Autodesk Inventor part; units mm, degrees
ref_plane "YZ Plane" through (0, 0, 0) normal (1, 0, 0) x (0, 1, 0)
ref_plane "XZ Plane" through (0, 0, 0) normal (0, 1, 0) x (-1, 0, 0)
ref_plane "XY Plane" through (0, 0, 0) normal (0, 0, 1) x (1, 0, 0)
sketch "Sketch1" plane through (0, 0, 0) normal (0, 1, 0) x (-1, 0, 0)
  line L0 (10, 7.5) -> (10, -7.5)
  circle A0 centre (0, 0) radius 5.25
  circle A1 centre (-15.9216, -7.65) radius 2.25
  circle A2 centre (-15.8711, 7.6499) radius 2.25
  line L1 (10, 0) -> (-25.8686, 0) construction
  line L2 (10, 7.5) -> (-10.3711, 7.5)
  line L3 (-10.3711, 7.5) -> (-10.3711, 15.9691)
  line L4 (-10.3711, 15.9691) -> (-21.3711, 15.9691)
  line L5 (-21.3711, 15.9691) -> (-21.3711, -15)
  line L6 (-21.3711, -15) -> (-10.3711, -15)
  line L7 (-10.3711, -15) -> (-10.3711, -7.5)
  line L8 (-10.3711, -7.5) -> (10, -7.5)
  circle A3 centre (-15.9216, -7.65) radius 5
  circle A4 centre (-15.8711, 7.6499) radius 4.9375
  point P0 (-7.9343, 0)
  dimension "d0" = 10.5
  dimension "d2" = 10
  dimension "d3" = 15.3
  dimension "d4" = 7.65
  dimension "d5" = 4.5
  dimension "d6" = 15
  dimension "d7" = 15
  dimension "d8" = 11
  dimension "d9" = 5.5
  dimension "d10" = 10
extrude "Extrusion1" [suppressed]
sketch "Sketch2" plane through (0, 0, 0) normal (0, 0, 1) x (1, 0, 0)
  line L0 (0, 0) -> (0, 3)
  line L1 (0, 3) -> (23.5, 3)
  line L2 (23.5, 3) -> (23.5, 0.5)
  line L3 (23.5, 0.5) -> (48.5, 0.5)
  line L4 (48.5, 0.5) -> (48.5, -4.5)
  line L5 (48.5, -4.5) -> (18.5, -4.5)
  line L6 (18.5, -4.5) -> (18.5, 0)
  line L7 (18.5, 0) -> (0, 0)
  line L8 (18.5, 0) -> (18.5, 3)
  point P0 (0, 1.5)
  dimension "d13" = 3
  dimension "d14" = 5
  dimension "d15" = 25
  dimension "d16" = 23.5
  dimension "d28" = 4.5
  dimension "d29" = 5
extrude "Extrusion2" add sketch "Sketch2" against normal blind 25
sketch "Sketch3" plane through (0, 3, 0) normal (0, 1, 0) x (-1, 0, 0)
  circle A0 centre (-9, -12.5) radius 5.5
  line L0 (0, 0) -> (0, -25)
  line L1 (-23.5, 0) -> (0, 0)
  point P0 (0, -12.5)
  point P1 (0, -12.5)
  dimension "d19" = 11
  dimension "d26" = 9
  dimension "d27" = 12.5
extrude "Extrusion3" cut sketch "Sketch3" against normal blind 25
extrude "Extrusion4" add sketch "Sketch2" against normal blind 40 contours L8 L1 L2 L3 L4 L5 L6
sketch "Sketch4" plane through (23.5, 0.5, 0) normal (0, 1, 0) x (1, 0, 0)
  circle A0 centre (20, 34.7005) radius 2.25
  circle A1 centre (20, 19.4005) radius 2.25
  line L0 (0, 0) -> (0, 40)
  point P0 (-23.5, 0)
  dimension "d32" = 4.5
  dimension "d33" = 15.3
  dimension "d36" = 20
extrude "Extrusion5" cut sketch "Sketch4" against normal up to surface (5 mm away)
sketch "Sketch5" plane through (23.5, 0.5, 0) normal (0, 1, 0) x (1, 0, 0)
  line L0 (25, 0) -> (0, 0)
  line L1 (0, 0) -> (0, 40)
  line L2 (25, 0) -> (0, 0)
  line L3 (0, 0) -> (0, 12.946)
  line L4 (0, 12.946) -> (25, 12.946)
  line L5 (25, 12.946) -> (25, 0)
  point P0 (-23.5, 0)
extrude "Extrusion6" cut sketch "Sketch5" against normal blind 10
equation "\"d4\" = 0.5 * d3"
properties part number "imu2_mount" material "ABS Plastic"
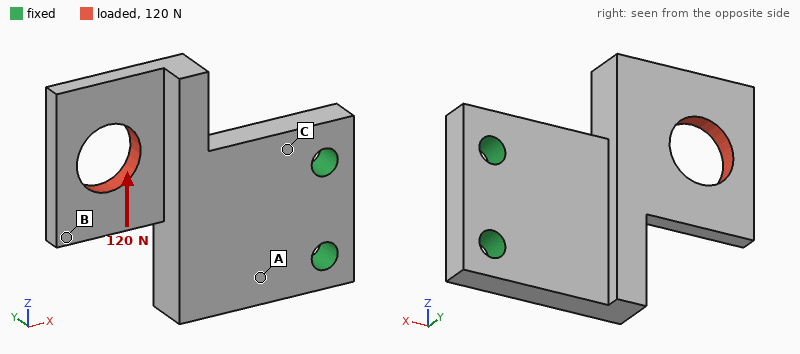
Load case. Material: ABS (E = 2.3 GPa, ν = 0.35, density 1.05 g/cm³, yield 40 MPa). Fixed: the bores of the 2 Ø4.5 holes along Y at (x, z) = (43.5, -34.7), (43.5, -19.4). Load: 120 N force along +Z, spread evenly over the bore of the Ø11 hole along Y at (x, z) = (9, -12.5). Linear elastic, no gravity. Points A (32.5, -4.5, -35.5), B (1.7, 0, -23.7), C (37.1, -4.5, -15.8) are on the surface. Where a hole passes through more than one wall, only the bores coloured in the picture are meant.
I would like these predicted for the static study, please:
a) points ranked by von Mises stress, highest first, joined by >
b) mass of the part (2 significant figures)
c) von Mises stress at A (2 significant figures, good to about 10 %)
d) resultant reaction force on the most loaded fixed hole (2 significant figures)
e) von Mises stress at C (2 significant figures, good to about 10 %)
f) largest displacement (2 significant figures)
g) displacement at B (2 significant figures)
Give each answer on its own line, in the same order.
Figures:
C > A > B
6.1 g
3.0 MPa
240 N
6.0 MPa
0.54 mm
0.42 mm
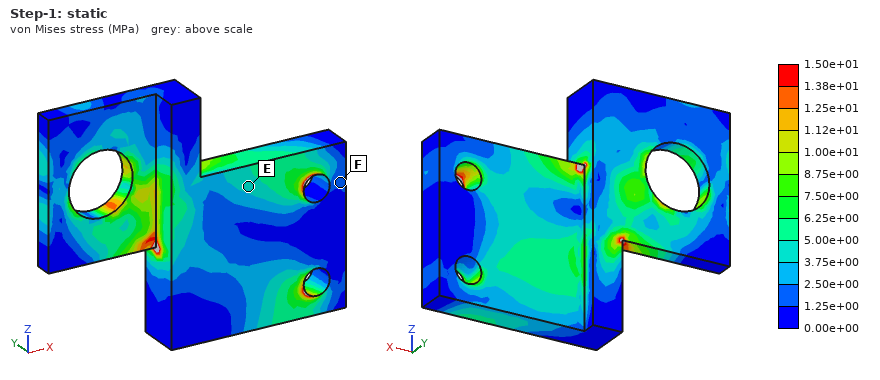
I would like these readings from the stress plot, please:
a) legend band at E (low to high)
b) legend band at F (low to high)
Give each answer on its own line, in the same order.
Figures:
3.75e+00 to 5.00e+00 MPa
1.25e+00 to 2.50e+00 MPa
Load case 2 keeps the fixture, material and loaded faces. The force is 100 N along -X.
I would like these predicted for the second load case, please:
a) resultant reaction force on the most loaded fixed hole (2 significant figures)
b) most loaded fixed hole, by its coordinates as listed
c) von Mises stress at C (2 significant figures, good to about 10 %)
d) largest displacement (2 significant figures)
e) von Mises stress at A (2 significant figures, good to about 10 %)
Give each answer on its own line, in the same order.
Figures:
130 N
(43.5, -19.4)
1.3 MPa
0.64 mm
3.2 MPa
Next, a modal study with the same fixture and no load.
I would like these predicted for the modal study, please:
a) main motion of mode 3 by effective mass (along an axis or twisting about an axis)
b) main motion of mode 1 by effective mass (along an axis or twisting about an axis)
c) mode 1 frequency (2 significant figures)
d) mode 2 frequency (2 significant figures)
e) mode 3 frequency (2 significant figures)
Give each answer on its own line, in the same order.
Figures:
along Z
along Y
730 Hz
1900 Hz
2200 Hz
